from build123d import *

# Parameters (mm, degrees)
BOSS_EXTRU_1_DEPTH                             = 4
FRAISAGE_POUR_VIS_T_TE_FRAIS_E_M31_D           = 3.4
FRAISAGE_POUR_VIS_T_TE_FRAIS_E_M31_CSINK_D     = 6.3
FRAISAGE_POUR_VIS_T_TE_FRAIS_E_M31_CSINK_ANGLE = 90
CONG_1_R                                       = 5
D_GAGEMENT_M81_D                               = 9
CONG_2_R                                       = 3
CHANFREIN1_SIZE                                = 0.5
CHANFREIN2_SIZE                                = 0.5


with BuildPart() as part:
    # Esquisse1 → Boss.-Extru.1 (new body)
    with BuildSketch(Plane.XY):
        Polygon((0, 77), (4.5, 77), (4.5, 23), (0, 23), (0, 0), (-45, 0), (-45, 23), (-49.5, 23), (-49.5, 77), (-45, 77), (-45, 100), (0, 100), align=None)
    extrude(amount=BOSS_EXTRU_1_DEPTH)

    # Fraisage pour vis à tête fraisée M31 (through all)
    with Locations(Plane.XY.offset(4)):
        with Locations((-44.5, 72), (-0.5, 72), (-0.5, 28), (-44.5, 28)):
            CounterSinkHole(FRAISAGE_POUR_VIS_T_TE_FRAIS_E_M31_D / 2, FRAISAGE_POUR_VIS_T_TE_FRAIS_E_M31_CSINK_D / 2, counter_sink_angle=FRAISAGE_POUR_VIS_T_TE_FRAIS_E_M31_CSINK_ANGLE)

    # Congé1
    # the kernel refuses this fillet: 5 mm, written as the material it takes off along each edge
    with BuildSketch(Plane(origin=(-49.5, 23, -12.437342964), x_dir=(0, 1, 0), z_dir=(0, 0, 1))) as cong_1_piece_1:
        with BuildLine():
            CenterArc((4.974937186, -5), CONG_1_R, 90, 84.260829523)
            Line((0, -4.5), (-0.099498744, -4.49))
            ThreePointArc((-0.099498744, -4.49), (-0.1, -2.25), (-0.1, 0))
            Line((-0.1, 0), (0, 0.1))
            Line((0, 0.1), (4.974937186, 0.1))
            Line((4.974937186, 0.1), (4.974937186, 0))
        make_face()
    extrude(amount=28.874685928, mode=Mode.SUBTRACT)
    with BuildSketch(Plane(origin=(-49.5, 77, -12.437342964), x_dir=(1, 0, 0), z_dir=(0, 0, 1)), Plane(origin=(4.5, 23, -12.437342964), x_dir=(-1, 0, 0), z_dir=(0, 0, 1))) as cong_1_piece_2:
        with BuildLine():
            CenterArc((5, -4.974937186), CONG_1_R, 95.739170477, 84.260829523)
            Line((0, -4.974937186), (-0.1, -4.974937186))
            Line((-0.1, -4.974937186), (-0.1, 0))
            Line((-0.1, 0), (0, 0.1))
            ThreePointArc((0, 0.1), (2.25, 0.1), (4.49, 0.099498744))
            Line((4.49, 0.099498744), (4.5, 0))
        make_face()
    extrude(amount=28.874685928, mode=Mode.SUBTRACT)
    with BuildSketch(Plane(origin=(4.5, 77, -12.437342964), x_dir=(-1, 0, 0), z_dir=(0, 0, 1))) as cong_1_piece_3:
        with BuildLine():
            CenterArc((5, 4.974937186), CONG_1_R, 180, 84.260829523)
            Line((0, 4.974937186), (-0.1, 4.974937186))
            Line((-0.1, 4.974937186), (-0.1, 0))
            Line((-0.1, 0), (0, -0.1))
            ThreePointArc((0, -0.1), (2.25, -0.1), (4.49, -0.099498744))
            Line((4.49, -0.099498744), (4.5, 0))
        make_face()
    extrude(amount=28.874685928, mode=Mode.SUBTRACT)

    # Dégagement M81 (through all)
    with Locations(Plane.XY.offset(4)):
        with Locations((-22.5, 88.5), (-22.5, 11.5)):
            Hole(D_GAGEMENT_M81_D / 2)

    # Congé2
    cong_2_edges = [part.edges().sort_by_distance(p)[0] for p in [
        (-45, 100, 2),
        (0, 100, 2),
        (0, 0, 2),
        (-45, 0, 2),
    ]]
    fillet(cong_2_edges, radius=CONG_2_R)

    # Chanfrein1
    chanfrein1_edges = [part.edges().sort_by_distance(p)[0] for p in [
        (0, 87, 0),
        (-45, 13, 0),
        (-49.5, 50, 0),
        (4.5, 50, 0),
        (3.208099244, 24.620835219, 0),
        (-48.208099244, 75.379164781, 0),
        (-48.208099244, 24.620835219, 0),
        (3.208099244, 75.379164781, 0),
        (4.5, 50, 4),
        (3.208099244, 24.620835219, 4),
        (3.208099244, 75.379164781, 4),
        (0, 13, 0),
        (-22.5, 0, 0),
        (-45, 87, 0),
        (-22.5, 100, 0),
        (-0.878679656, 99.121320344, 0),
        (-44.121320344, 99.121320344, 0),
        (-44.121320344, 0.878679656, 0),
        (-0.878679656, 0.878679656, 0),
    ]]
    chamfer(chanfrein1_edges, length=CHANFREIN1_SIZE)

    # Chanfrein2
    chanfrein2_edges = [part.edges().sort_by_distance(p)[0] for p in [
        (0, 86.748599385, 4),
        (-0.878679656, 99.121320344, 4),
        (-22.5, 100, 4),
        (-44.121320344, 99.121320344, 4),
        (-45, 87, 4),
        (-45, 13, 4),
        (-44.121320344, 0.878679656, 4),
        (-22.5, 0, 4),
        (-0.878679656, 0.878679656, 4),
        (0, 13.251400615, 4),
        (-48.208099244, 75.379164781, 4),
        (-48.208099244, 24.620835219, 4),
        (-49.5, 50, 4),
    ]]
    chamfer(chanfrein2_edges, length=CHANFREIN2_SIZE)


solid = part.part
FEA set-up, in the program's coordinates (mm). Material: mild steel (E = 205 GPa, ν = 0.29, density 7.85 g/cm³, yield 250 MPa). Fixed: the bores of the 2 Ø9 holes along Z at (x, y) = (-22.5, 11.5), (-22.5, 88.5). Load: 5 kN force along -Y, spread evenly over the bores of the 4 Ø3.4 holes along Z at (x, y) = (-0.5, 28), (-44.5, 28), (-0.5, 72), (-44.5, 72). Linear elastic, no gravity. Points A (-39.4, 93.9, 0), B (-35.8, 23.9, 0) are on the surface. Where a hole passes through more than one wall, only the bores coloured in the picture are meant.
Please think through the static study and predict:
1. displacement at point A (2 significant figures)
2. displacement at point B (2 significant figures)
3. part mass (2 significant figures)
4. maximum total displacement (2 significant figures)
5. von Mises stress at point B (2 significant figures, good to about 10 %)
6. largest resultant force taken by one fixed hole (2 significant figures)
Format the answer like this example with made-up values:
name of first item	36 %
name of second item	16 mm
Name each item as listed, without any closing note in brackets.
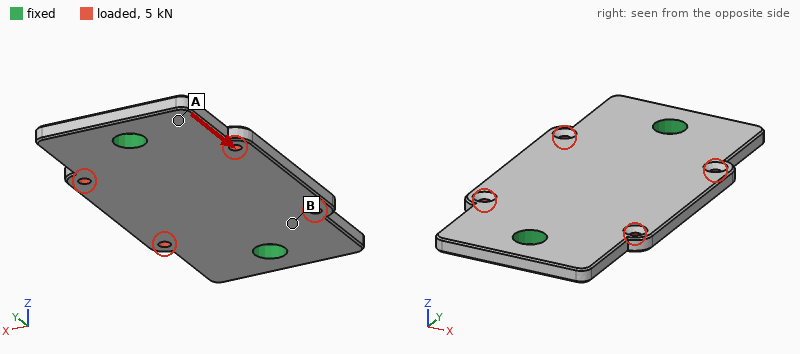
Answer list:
displacement at point A	2.0 µm
displacement at point B	2.1 µm
part mass	150 g
maximum total displacement	4.7 µm
von Mises stress at point B	20 MPa
largest resultant force taken by one fixed hole	2.5 kN
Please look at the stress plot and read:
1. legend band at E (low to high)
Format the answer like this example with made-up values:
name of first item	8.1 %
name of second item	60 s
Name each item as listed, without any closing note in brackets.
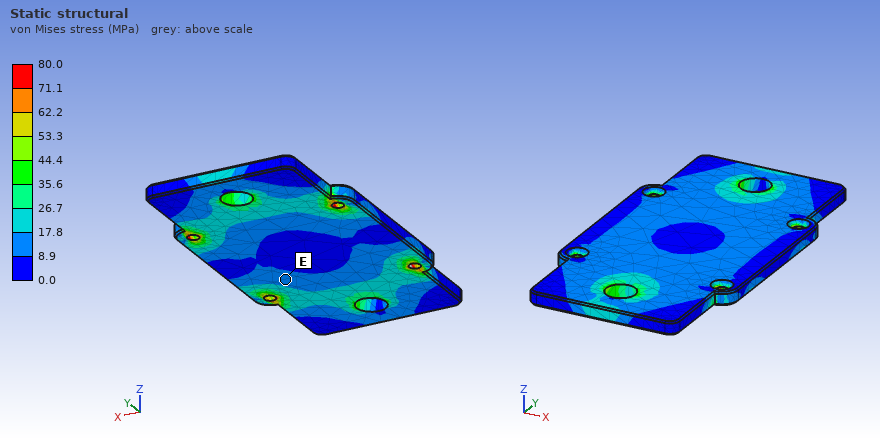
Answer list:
legend band at E	8.9 to 17.8 MPa
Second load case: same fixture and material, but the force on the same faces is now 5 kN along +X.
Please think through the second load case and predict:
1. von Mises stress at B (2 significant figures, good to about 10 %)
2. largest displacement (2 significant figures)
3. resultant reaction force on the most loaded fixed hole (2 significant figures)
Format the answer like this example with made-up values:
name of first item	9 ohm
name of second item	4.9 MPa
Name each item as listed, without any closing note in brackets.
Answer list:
von Mises stress at B	36 MPa
largest displacement	14 µm
resultant reaction force on the most loaded fixed hole	2.5 kN
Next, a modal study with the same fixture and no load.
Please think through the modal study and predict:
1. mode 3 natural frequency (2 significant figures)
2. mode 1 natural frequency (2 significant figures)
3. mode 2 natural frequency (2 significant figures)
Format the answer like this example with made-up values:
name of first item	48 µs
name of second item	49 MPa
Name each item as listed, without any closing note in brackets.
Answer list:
mode 3 natural frequency	7100 Hz
mode 1 natural frequency	3100 Hz
mode 2 natural frequency	3200 Hz
